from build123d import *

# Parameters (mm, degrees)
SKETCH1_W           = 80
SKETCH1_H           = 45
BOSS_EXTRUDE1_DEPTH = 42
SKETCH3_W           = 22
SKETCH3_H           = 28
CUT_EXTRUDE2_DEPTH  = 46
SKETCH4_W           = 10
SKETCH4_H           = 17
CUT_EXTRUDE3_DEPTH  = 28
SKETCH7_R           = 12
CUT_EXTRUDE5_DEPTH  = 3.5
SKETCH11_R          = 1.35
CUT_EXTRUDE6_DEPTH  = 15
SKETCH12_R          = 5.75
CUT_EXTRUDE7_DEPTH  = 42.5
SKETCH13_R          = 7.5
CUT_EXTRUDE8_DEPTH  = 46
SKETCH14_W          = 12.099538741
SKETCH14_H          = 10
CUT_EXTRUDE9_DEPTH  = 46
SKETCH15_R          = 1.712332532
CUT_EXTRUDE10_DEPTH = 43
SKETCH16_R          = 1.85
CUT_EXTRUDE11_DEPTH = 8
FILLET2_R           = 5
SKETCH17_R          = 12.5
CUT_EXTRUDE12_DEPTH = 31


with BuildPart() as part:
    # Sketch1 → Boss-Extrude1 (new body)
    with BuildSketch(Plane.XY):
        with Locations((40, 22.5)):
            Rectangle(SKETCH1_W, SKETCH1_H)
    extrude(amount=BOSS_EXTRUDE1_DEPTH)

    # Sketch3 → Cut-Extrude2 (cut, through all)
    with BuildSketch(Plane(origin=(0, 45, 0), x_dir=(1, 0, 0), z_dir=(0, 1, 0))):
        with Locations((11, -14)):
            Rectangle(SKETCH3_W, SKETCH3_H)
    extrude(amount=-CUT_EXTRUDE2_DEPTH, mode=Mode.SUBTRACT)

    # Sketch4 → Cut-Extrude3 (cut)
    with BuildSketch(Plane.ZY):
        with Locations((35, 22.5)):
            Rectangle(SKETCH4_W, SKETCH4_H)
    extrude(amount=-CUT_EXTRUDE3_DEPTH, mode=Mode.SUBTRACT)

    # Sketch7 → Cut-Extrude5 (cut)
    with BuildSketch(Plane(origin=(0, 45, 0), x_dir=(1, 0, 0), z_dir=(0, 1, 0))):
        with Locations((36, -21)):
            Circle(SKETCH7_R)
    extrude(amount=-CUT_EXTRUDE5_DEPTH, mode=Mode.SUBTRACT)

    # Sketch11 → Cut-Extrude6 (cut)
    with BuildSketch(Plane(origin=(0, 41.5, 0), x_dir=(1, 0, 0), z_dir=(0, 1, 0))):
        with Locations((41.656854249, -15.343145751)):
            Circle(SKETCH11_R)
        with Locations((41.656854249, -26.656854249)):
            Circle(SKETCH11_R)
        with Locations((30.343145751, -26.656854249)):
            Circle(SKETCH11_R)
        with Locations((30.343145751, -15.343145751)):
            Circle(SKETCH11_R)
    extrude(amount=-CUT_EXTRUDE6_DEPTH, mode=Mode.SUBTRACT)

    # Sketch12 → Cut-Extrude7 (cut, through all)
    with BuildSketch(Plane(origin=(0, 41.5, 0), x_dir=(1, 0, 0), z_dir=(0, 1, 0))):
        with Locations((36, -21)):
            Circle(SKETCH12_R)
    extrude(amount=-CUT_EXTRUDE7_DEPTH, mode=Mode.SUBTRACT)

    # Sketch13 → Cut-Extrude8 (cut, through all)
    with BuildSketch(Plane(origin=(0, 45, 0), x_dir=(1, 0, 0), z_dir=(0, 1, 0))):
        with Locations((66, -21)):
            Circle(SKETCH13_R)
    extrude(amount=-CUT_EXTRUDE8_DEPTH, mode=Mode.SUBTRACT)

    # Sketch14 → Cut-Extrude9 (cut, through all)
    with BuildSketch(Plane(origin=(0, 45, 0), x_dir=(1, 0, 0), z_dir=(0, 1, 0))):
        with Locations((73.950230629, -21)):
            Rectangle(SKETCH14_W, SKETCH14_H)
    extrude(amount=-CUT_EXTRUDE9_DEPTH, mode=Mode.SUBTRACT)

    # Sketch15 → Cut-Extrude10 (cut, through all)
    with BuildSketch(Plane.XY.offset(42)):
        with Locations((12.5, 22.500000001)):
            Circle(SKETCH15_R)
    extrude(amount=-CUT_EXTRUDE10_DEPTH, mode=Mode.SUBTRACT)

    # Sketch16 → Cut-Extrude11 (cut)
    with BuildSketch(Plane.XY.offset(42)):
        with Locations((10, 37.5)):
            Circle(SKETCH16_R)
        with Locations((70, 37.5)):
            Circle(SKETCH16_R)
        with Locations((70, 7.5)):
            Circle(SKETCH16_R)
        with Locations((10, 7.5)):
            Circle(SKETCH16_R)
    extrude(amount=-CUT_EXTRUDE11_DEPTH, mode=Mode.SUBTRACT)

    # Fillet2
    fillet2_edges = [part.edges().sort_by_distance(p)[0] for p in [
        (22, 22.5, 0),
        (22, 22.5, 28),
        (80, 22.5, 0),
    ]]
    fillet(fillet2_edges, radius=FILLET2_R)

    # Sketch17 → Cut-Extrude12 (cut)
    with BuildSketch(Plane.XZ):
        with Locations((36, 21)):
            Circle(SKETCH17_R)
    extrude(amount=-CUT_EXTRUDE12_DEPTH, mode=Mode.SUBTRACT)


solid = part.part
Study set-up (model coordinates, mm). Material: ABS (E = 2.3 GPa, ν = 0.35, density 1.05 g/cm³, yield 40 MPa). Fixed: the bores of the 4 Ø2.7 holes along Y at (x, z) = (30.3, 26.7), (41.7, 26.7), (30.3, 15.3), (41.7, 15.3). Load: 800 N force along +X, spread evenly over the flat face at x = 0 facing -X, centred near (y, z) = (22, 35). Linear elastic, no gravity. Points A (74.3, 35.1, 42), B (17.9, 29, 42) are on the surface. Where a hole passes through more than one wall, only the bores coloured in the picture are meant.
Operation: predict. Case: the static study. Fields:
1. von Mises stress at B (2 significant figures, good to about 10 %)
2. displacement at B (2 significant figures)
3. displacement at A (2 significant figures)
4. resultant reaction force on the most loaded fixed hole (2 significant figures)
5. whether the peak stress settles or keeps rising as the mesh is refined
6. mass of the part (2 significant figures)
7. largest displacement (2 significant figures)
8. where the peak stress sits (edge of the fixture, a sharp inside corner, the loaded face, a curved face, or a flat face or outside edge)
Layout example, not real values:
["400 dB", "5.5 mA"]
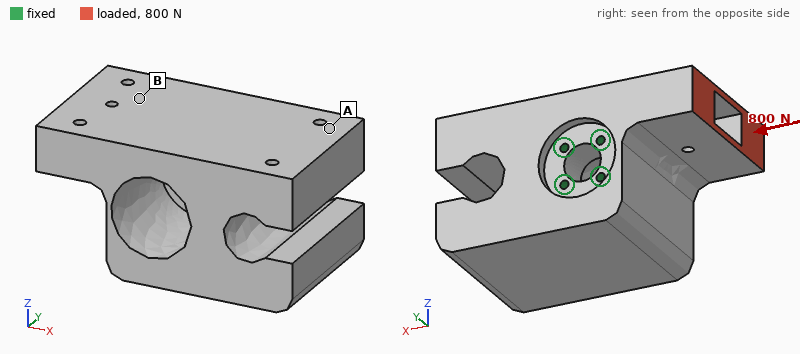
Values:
["2.9 MPa", "0.11 mm", "0.17 mm", "590 N", "keeps rising", "93 g", "0.28 mm", "edge of the fixture"]
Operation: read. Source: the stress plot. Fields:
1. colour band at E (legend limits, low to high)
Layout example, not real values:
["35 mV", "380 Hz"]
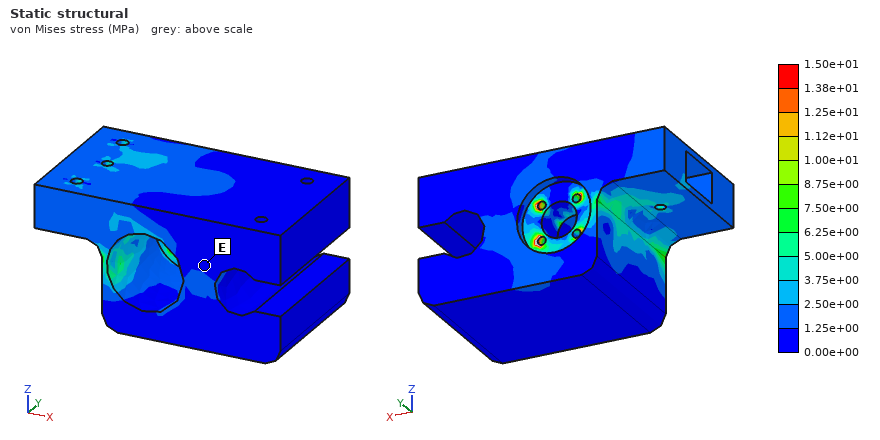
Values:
["0.00e+00 to 1.25e+00 MPa"]
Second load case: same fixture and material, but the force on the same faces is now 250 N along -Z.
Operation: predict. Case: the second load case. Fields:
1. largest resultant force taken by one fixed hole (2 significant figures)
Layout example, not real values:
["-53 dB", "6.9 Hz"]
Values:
["350 N"]
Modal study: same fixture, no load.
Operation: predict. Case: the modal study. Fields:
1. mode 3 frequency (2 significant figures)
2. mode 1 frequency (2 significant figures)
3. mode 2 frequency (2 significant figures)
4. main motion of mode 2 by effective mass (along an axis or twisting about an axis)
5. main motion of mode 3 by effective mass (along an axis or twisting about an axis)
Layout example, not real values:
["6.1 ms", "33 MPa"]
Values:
["1600 Hz", "990 Hz", "1200 Hz", "along Z", "twisting about Y"]
